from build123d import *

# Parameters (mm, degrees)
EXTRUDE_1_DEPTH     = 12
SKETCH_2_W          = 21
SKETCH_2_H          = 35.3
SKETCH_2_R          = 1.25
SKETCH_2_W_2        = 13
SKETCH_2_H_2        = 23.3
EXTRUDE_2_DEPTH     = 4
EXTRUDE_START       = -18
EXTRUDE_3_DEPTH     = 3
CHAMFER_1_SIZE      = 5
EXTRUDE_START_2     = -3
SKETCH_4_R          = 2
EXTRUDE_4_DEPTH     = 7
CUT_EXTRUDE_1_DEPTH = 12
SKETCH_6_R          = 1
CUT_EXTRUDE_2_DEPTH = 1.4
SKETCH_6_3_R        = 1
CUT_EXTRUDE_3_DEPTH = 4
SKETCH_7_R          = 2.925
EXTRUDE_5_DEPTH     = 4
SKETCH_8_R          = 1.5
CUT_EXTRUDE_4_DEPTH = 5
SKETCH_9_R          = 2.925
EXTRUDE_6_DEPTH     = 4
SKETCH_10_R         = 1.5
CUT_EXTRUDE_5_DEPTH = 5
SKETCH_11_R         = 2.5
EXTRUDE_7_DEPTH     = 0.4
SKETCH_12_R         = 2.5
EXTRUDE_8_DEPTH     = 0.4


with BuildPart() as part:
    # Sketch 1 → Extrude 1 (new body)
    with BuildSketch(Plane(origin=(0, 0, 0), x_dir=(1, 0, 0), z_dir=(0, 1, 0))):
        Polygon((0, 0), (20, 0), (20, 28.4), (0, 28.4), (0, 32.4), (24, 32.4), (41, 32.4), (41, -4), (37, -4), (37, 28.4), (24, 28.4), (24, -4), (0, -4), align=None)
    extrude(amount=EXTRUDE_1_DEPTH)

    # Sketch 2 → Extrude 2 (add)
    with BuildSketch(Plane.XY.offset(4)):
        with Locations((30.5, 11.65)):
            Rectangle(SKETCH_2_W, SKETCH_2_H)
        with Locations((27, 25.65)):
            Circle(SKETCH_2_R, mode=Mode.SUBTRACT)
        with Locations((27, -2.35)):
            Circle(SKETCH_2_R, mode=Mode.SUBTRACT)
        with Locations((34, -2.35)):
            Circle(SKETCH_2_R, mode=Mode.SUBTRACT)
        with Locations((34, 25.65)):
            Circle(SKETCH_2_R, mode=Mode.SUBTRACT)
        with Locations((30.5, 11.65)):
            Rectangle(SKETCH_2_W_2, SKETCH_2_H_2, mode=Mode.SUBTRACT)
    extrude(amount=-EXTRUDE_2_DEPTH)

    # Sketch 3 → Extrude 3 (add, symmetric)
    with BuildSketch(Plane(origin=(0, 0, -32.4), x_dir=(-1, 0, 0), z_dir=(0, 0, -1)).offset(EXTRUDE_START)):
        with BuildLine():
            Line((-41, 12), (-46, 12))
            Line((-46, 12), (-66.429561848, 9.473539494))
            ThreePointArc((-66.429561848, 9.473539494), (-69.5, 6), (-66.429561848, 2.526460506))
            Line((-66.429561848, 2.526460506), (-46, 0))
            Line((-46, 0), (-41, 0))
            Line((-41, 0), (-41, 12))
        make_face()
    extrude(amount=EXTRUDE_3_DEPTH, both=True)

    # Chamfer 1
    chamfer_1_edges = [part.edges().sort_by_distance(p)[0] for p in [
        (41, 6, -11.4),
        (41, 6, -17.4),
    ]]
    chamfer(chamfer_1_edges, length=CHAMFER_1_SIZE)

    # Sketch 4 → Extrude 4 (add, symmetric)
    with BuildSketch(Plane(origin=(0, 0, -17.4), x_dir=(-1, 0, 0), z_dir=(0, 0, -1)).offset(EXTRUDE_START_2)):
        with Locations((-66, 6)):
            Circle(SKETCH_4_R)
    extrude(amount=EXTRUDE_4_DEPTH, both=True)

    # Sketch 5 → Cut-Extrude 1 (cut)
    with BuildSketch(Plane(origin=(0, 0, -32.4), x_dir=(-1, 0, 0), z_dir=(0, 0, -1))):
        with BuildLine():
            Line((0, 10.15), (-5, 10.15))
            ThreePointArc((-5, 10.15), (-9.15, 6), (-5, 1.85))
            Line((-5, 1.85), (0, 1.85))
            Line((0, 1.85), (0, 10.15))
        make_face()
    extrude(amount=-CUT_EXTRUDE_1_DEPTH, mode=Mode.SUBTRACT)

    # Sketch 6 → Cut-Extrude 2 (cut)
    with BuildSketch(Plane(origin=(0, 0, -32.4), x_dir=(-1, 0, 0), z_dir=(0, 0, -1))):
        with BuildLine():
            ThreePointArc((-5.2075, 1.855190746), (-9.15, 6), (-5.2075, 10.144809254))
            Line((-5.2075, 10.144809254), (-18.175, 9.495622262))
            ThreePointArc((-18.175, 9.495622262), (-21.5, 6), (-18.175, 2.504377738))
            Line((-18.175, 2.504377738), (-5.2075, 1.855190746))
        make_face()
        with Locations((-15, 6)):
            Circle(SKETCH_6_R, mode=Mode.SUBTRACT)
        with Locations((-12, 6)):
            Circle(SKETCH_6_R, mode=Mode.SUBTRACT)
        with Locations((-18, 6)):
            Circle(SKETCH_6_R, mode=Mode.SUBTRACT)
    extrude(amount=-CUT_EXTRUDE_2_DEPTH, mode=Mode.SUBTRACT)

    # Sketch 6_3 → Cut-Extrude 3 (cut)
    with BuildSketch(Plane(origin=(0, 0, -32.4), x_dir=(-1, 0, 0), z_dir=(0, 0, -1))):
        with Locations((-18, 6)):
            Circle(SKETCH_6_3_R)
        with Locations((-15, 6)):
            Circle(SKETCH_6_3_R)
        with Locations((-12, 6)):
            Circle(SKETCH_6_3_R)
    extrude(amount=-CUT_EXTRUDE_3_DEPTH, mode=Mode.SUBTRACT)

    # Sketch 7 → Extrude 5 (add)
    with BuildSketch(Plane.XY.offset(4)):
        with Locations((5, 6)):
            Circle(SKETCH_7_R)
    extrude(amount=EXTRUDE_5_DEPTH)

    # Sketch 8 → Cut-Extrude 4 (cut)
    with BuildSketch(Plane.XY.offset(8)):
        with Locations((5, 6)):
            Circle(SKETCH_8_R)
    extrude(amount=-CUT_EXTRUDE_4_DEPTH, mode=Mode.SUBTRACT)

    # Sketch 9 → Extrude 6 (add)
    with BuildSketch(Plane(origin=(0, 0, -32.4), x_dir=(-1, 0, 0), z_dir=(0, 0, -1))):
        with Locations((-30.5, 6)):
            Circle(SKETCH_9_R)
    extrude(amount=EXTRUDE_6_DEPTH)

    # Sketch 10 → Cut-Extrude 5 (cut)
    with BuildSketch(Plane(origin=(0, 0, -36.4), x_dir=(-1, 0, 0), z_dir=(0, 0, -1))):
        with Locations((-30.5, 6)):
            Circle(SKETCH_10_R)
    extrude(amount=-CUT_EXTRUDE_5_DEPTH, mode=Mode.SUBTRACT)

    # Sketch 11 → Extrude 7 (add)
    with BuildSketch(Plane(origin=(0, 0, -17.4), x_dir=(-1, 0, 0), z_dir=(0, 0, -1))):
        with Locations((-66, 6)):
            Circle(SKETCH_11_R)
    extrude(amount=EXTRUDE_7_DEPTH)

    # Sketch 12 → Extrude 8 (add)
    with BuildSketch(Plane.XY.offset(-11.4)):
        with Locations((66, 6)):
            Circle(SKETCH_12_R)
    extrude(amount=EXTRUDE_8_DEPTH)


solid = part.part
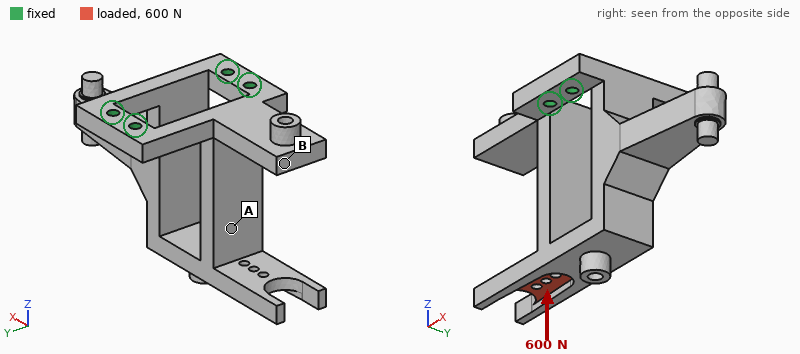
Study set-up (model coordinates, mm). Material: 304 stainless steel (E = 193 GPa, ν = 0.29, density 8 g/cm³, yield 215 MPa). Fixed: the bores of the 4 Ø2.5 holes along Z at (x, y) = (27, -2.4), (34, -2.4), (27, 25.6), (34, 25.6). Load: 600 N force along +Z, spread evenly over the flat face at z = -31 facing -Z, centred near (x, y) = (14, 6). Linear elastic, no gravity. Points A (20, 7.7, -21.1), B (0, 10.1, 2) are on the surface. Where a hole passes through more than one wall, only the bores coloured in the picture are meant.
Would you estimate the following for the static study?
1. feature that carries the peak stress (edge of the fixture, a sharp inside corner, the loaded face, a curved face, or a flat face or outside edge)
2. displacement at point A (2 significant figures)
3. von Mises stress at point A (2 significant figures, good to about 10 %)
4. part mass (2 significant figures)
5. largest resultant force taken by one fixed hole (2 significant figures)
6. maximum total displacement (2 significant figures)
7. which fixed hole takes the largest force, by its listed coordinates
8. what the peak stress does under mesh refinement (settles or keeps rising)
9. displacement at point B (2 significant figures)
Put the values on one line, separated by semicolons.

edge of the fixture; 0.032 mm; 45 MPa; 73 g; 720 N; 0.13 mm; (27, -2.4); keeps rising; 0.036 mm
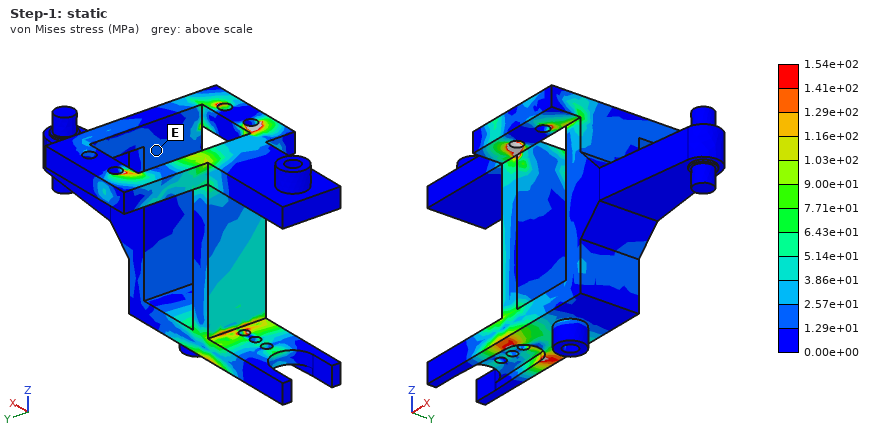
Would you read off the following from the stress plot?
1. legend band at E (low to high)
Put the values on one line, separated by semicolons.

1.29e+01 to 2.57e+01 MPa
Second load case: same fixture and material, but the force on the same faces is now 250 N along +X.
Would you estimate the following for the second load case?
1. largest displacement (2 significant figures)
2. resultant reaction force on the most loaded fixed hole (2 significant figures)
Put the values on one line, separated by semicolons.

0.11 mm; 320 N
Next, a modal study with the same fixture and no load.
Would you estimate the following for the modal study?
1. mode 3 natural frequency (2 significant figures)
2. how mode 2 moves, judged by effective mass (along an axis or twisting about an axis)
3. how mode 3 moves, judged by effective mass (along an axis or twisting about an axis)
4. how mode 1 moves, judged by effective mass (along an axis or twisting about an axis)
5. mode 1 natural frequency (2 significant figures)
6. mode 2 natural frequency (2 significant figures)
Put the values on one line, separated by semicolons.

2700 Hz; along Y; twisting about Z; along X; 1500 Hz; 2400 Hz
